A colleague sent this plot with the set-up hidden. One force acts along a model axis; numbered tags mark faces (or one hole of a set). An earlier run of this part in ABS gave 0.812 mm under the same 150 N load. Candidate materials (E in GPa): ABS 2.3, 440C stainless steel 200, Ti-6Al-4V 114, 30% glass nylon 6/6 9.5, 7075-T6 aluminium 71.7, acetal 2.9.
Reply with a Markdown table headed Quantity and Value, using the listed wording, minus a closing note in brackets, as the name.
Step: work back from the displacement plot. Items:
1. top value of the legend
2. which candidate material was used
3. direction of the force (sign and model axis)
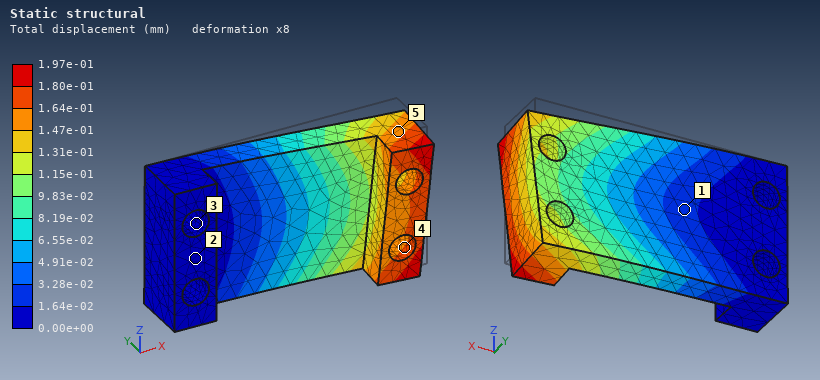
| Quantity | Value |
|---|---|
| top value of the legend | 1.97e-01 mm |
| which candidate material was used | 30% glass nylon 6/6 |
| direction of the force | -Z |
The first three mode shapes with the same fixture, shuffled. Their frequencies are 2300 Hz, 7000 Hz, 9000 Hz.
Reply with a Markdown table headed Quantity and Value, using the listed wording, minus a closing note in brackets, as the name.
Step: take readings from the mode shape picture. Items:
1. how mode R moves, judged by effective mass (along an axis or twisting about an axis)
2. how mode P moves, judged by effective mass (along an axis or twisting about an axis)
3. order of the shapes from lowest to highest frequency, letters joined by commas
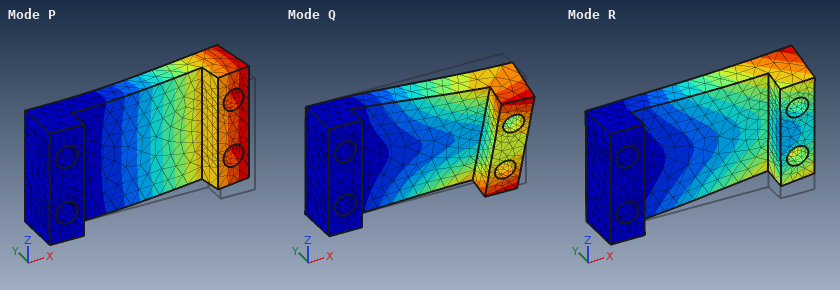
| Quantity | Value |
|---|---|
| how mode R moves, judged by effective mass | along Z |
| how mode P moves, judged by effective mass | along Y |
| order of the shapes from lowest to highest frequency, letters joined by commas | P, Q, R |
